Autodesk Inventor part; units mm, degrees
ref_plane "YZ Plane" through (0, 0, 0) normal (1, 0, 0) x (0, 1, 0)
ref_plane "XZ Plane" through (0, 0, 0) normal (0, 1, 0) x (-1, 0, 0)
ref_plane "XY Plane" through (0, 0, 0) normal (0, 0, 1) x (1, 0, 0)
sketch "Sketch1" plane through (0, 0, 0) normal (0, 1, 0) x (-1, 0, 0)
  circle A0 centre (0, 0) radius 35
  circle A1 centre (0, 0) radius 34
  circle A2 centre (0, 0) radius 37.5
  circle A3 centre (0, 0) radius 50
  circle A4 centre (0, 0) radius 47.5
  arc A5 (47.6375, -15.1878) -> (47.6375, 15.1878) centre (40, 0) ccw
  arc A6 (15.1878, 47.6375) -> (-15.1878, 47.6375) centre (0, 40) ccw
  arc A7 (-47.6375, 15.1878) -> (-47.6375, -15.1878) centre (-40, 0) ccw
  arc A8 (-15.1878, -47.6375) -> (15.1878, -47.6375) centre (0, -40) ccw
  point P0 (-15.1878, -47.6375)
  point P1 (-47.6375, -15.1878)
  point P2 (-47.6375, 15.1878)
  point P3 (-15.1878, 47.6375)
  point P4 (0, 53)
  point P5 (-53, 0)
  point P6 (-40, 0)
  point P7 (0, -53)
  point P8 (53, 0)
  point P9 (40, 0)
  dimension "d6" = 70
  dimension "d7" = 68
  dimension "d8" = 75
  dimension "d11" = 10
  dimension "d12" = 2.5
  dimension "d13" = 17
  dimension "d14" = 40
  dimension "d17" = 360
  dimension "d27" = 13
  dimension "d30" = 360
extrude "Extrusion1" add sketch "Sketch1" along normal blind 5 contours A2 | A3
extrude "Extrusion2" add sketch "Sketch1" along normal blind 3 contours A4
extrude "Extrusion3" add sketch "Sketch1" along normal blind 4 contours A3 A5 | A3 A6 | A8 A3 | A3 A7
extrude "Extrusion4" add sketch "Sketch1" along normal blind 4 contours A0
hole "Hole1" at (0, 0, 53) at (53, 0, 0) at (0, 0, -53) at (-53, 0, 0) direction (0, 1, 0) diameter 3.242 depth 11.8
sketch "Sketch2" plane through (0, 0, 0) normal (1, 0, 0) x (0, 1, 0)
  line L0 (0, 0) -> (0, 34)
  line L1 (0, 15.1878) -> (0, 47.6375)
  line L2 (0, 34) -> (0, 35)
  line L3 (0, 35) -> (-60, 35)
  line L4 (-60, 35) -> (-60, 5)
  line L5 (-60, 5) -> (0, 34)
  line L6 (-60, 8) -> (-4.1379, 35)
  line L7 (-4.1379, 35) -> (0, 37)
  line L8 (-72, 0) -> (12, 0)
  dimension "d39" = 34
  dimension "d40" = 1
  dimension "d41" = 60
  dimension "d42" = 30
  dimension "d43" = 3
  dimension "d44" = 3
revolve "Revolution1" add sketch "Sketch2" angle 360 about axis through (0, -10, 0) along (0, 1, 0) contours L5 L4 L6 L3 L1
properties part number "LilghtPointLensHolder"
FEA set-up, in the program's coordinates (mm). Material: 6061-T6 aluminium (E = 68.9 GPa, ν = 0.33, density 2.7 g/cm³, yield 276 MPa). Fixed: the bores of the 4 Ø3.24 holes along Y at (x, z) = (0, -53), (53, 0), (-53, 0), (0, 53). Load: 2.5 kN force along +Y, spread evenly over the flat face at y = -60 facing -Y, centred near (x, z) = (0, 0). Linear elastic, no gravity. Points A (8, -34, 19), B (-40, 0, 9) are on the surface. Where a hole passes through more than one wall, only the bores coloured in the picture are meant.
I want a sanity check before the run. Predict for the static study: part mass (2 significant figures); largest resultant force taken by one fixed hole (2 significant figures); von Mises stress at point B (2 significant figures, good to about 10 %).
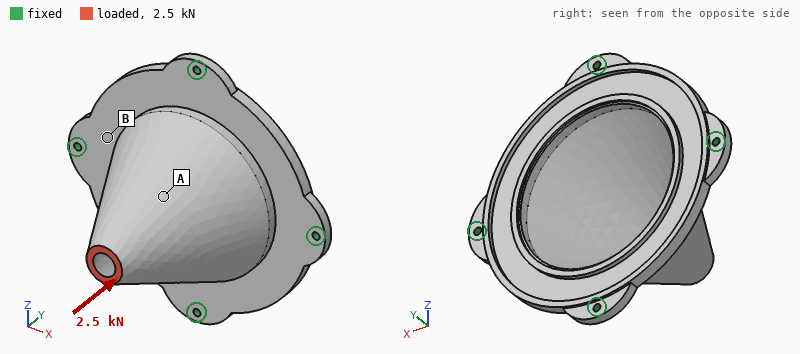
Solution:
110 g
790 N
31 MPa
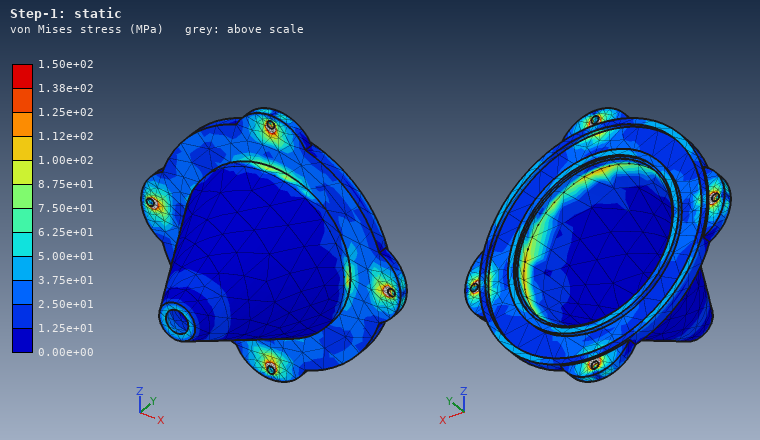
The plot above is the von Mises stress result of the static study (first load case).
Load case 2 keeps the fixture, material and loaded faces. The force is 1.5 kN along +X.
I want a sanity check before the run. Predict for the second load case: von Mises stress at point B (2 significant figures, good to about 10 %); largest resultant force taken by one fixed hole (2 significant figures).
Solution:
60 MPa
1.3 kN
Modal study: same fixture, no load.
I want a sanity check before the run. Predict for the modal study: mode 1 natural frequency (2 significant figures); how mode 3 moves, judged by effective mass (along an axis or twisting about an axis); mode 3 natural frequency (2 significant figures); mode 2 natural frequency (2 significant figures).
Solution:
2400 Hz
along Y
2600 Hz
2400 Hz
